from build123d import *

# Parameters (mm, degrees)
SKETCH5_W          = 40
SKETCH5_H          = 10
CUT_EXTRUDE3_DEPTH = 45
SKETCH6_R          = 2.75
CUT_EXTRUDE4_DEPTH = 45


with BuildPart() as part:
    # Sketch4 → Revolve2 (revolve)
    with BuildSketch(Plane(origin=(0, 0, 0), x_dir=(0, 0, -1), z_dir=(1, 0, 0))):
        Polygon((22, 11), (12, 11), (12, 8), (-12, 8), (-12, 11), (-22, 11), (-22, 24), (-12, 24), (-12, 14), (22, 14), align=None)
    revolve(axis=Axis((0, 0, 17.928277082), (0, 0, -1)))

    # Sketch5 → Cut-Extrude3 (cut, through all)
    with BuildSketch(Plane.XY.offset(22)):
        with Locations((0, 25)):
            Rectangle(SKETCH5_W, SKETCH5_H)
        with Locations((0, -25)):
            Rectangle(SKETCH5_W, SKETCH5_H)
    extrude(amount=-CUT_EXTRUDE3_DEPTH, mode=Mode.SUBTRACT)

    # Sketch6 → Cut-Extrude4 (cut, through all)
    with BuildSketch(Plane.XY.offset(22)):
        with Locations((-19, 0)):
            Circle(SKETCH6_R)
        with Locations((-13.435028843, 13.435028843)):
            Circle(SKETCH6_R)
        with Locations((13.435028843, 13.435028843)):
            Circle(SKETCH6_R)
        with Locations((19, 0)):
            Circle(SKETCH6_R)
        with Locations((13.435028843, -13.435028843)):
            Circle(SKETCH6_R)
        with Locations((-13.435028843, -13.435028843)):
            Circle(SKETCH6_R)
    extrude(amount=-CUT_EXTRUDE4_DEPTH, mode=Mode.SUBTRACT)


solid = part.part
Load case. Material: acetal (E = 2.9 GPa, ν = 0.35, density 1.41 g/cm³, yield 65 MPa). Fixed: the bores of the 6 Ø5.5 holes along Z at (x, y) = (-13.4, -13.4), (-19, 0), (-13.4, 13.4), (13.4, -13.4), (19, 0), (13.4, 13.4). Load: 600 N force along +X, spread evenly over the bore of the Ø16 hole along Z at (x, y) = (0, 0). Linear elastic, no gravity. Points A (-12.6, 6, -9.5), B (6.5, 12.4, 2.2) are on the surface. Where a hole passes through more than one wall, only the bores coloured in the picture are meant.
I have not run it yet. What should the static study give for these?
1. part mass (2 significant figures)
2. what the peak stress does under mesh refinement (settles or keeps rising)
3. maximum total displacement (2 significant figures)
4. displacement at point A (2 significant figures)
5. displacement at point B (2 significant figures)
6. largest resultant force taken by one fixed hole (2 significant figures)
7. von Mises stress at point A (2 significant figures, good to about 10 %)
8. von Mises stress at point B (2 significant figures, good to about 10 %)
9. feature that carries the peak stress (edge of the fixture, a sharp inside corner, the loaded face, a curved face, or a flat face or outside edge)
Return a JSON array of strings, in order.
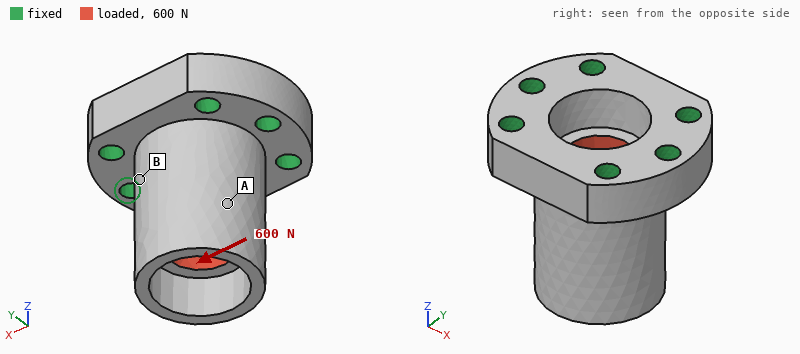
["33 g", "keeps rising", "69 µm", "56 µm", "30 µm", "190 N", "0.75 MPa", "1.9 MPa", "a sharp inside corner"]
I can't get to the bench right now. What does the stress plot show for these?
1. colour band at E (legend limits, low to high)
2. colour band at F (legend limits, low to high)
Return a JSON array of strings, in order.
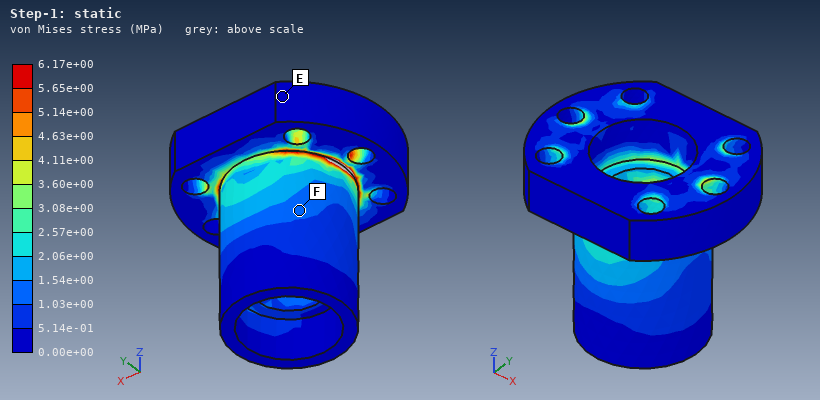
["0.00e+00 to 5.14e-01 MPa", "1.03e+00 to 1.54e+00 MPa"]
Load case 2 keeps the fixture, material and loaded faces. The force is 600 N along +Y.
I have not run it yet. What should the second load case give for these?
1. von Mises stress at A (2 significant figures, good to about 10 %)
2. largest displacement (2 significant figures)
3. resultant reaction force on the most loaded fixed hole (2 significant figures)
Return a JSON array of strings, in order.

["0.63 MPa", "85 µm", "220 N"]
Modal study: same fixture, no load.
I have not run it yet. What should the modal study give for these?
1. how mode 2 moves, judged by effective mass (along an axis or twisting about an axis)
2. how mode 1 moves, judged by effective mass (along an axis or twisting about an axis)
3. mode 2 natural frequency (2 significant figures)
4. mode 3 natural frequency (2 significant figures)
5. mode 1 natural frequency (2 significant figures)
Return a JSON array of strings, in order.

["along X", "along Y", "3600 Hz", "5900 Hz", "3300 Hz"]
